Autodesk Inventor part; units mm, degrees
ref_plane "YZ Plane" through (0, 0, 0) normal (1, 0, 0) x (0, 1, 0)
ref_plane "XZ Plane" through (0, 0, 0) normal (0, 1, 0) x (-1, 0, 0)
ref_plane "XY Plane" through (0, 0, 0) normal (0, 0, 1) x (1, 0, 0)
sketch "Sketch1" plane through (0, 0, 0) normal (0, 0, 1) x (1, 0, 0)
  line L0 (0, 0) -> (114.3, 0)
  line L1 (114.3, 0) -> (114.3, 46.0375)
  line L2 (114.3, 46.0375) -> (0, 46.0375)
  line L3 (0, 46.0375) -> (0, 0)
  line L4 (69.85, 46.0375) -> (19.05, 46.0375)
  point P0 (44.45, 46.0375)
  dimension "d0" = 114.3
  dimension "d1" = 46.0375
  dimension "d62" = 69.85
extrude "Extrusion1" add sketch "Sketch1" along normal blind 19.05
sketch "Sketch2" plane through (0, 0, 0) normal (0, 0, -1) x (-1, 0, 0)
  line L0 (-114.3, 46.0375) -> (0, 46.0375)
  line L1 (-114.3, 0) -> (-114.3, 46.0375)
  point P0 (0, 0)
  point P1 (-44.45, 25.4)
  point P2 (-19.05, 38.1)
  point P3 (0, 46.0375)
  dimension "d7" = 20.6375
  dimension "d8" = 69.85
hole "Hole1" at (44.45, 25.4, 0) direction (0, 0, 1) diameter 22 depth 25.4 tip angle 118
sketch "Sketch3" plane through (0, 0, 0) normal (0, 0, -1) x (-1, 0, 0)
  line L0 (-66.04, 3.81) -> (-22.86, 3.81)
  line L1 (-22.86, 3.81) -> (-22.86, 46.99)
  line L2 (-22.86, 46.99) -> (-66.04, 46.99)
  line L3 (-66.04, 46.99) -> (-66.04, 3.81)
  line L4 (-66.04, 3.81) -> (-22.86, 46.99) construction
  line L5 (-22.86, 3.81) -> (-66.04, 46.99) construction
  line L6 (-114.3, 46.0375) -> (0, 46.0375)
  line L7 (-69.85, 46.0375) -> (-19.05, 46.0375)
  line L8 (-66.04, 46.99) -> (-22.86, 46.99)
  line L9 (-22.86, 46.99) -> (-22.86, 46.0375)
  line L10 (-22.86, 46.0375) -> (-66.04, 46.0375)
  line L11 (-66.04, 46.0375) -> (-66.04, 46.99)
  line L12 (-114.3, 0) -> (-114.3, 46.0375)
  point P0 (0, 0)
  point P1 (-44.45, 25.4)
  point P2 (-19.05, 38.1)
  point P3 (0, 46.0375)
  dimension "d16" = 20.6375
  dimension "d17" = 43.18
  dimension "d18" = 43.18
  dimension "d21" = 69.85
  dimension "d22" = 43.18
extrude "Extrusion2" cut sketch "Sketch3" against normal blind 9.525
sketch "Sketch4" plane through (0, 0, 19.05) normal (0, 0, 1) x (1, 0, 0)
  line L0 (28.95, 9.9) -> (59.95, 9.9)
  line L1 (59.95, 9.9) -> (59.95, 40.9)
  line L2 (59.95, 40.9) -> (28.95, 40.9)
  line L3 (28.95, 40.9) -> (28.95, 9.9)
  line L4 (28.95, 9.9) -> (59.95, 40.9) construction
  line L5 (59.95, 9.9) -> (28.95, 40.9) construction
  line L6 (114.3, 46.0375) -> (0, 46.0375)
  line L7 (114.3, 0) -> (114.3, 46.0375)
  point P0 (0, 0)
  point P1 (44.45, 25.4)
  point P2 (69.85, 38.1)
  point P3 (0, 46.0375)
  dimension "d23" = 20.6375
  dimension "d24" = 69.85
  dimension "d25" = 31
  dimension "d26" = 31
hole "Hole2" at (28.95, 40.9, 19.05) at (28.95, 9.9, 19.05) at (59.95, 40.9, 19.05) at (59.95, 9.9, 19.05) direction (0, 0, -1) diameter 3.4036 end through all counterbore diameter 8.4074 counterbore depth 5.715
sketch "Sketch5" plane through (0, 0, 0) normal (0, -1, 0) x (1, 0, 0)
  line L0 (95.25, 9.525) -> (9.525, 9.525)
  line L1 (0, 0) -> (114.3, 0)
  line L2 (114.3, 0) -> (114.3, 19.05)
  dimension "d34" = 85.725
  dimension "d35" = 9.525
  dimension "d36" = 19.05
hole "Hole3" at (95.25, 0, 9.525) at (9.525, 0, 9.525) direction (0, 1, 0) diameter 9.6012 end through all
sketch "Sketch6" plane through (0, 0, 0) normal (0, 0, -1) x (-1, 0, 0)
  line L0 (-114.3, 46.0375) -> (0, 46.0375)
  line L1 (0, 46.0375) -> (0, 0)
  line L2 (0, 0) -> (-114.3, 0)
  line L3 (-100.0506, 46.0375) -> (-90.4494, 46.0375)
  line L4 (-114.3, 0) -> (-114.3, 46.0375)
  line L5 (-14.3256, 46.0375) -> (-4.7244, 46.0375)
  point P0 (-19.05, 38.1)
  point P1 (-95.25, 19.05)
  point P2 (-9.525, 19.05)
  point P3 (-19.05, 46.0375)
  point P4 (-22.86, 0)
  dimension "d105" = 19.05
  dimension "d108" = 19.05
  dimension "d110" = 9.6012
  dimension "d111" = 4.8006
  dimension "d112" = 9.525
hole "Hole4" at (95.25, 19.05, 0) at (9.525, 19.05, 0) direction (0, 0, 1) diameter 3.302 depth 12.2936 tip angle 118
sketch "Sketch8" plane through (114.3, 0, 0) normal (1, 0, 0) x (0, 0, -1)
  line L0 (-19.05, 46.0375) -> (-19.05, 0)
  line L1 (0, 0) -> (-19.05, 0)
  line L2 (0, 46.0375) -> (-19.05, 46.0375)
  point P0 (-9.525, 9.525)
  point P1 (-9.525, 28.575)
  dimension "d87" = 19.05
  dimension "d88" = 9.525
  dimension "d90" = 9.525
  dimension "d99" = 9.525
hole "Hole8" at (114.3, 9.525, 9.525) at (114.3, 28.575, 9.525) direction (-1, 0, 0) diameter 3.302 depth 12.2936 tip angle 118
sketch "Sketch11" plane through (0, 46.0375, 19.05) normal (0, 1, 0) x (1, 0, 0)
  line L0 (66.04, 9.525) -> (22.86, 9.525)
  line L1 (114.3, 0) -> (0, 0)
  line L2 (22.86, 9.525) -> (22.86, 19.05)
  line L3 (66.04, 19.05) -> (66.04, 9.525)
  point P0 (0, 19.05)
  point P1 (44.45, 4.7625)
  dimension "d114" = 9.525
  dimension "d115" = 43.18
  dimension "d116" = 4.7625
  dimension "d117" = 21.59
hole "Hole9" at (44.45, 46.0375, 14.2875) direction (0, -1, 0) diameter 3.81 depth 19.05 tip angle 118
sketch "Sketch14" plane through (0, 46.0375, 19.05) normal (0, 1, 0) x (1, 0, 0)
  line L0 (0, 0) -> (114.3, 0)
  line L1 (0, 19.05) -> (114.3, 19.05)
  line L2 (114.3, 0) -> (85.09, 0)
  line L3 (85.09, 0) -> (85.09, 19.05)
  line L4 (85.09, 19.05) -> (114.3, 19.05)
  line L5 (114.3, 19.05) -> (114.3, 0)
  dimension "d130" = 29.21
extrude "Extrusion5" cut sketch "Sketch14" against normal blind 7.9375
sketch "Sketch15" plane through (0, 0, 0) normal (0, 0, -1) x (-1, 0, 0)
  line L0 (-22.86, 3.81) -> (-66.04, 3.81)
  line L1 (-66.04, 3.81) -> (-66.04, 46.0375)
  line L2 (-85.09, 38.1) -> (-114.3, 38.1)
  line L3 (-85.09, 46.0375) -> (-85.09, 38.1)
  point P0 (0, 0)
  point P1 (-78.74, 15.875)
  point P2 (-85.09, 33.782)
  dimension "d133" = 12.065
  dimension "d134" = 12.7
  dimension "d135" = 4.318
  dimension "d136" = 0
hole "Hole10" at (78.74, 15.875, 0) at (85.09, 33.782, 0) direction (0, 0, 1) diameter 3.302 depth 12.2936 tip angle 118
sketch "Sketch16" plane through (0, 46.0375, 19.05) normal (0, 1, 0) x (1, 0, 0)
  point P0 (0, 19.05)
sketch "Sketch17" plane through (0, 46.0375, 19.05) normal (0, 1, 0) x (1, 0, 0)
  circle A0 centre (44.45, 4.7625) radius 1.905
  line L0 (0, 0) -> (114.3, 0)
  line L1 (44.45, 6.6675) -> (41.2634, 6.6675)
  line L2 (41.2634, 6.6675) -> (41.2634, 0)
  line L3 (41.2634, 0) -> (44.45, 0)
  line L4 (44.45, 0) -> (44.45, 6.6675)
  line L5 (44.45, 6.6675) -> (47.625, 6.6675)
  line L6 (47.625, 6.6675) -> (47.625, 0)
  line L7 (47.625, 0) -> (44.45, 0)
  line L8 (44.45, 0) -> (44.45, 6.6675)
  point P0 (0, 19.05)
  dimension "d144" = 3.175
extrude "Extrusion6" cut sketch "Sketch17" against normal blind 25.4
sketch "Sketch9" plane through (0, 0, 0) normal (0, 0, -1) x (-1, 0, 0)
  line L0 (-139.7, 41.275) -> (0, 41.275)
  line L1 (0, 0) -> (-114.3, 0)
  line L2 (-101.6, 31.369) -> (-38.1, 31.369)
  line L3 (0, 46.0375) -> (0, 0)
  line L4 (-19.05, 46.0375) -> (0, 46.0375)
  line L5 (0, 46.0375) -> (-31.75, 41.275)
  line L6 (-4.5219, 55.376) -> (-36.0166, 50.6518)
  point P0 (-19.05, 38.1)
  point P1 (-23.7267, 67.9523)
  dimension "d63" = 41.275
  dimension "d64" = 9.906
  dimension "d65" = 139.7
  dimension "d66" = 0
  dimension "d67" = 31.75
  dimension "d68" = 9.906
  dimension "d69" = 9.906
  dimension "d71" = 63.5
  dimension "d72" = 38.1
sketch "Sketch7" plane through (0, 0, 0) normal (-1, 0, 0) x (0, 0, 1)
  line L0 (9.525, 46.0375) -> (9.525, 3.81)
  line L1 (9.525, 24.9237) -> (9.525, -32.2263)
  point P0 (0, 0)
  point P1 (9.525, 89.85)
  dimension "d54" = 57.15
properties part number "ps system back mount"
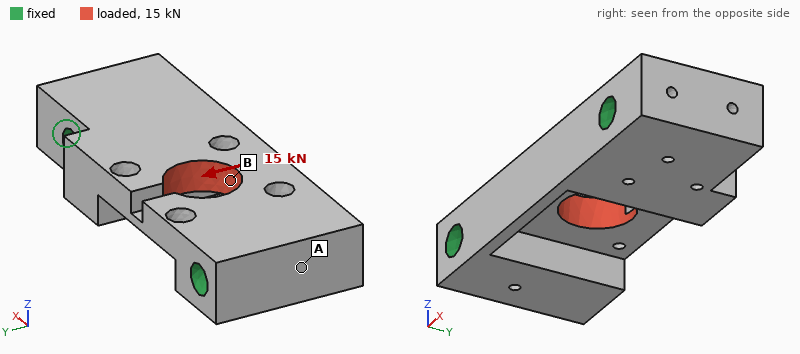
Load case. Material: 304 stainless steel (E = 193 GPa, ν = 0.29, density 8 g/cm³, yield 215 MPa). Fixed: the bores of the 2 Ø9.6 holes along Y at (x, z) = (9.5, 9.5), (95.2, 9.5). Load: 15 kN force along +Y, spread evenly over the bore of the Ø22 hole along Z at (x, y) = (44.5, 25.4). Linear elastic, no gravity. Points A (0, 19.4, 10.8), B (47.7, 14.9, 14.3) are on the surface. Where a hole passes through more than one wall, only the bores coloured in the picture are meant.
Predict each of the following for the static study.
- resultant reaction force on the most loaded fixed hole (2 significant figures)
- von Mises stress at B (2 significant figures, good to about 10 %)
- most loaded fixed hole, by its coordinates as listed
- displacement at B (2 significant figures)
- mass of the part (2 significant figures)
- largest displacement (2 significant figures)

8.8 kN
24 MPa
(9.5, 9.5)
12 µm
530 g
18 µm
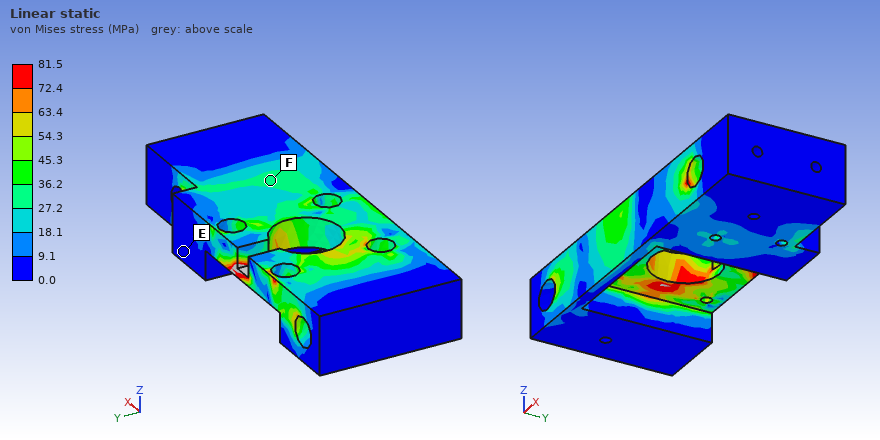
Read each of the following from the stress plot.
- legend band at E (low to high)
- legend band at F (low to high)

0.0 to 9.1 MPa
27.2 to 36.2 MPa
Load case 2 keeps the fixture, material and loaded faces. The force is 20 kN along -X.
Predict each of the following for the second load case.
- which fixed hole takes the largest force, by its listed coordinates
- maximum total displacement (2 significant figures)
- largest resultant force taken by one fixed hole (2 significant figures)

(9.5, 9.5)
7.5 µm
11 kN
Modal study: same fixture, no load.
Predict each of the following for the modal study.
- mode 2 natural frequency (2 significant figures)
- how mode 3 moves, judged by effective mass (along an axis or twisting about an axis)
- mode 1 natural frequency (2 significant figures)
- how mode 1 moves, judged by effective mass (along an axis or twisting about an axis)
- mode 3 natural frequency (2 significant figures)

13 kHz
along Y
9300 Hz
along Z
15 kHz
